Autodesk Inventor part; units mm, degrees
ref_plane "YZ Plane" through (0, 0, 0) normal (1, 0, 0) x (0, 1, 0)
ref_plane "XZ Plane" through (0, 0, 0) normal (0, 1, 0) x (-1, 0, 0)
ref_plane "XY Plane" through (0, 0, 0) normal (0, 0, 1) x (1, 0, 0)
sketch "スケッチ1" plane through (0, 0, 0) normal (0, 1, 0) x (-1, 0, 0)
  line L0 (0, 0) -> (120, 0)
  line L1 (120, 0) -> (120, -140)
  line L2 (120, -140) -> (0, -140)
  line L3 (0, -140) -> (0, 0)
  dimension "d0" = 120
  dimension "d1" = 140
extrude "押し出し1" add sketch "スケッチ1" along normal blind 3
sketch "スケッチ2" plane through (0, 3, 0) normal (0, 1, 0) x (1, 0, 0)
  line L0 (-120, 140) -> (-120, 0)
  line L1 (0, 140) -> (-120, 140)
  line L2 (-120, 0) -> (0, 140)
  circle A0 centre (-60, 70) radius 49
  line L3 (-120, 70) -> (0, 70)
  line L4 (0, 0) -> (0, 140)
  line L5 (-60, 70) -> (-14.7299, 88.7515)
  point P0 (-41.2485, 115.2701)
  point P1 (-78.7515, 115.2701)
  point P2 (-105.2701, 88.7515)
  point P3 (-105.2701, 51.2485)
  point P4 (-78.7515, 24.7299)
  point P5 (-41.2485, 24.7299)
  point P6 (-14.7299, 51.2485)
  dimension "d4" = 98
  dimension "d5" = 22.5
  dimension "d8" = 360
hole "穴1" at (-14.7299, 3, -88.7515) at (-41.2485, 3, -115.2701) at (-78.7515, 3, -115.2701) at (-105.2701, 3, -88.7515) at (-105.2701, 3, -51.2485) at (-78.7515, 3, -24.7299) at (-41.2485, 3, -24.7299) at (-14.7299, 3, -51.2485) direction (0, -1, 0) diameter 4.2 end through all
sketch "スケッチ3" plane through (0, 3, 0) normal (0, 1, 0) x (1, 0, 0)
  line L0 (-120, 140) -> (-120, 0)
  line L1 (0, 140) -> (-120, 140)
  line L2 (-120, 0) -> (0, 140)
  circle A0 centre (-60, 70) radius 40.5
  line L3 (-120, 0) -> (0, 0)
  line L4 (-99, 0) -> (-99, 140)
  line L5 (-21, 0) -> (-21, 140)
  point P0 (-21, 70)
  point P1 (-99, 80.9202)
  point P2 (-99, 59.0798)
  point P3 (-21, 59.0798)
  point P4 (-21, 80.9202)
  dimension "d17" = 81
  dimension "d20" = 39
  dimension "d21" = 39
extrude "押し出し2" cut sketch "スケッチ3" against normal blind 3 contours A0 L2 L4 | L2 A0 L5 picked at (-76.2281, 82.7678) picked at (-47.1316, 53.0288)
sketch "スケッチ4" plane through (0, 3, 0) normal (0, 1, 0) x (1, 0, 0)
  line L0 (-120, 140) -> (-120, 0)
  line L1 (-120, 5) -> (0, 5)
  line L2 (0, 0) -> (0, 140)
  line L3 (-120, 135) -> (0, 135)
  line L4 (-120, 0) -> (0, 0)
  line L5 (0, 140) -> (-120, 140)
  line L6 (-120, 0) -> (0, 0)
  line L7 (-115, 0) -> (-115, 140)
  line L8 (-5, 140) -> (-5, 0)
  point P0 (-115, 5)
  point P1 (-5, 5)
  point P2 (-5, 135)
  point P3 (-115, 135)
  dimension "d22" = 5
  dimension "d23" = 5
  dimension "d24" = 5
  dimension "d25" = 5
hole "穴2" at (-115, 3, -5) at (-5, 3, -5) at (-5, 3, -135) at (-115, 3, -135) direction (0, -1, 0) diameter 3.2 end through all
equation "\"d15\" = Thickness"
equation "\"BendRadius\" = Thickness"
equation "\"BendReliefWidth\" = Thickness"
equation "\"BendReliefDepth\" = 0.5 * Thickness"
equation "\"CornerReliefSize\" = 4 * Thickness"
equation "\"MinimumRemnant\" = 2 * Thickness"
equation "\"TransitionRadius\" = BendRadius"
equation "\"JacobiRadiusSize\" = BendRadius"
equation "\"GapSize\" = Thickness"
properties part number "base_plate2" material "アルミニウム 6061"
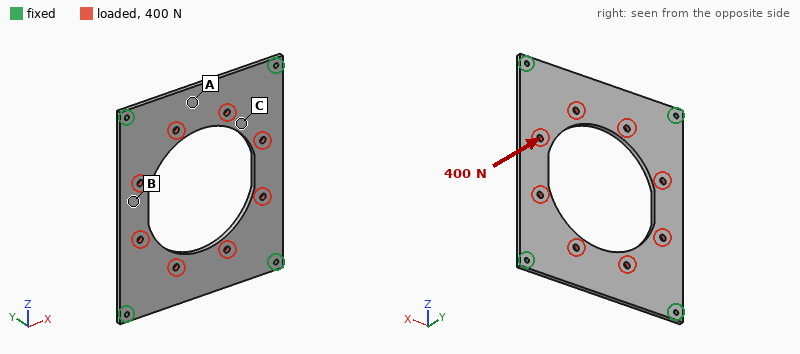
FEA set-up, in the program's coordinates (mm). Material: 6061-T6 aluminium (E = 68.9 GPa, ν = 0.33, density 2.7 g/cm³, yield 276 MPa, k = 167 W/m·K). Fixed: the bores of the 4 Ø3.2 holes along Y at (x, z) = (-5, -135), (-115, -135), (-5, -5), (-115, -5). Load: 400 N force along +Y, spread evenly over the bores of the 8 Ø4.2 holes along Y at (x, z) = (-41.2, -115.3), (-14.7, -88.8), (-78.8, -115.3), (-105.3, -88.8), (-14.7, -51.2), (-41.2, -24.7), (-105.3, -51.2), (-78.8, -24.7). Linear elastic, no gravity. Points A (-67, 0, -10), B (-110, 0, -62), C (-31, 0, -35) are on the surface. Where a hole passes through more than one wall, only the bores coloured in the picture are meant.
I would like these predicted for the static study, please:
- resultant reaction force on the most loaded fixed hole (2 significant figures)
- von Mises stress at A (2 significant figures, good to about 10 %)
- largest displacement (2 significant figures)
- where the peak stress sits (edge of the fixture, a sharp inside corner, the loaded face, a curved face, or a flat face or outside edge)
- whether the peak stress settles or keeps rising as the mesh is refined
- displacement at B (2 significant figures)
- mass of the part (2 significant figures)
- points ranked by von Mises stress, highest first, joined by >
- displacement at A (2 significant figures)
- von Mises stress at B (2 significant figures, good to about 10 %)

100 N
18 MPa
0.47 mm
edge of the fixture
keeps rising
0.38 mm
94 g
B > A > C
0.18 mm
32 MPa
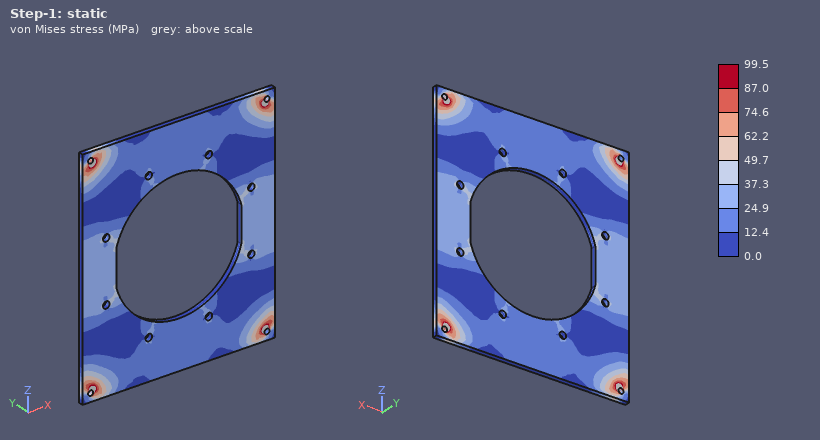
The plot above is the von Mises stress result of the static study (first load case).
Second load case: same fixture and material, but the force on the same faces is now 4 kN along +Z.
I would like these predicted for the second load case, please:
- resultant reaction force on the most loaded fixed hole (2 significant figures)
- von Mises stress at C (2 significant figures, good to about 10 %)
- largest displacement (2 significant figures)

1.1 kN
7.9 MPa
23 µm
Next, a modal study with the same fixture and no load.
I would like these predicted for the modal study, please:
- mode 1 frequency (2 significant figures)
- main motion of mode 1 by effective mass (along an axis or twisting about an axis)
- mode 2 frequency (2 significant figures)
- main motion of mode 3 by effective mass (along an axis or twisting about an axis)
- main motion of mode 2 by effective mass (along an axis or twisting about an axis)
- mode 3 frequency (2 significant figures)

760 Hz
along Y
1000 Hz
twisting about X
twisting about Z
1200 Hz
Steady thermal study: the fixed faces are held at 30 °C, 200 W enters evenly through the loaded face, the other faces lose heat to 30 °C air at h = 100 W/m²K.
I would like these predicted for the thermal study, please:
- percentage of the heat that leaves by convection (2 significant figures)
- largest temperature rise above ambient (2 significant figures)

59 %
76 K
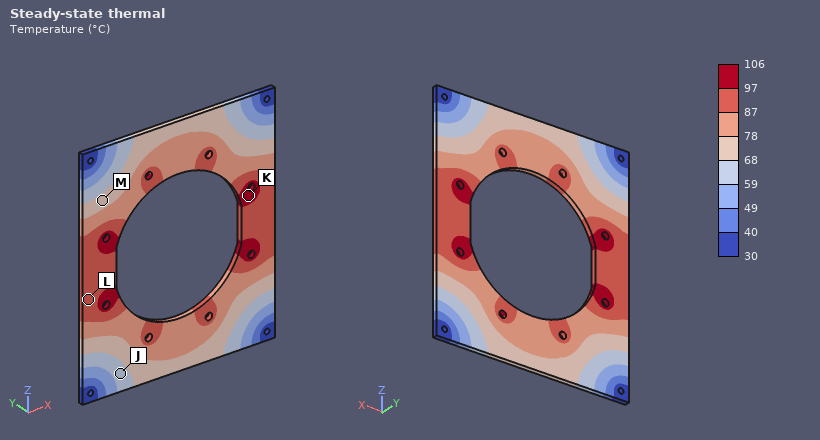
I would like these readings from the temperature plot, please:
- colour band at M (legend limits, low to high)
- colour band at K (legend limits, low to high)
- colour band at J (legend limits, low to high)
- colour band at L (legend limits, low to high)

68 to 78 °C
97 to 106 °C
59 to 68 °C
87 to 97 °C
